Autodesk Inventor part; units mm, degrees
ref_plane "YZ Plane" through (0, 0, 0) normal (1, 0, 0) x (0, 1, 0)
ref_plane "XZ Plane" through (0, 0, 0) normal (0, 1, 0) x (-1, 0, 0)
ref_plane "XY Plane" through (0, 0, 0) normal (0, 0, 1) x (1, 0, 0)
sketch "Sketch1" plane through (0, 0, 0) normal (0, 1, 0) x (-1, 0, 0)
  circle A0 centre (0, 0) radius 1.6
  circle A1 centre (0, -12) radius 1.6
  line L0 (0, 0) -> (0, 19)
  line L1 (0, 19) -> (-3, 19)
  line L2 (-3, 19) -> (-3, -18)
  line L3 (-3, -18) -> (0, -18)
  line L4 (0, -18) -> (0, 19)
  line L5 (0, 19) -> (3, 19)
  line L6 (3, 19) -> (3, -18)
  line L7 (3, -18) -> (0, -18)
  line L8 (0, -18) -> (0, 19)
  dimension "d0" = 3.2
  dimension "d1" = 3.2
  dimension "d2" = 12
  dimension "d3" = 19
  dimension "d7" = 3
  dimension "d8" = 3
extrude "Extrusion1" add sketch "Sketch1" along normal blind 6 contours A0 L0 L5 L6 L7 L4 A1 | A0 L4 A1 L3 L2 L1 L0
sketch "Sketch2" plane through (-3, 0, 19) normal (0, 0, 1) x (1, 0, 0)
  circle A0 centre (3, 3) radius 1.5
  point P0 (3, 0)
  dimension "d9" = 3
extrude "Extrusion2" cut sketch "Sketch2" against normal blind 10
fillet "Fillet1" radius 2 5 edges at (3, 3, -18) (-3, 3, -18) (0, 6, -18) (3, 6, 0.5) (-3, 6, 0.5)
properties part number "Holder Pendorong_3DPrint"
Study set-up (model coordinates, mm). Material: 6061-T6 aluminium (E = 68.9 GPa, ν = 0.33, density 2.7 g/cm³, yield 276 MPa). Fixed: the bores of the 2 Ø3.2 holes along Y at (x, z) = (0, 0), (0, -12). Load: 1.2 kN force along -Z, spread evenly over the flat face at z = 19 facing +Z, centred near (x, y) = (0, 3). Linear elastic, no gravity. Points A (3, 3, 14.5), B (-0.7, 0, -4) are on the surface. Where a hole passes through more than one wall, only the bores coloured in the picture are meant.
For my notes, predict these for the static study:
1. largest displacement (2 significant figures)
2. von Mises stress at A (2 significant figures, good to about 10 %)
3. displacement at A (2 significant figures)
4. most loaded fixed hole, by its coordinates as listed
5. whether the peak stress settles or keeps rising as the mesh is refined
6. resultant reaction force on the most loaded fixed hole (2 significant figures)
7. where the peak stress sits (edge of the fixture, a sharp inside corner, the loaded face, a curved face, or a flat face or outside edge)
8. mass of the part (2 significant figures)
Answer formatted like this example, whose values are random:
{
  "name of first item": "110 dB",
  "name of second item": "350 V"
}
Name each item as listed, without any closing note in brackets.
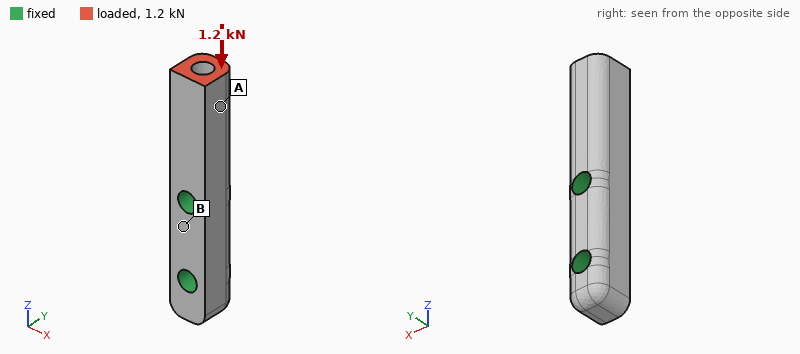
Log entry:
{
  "largest displacement": "11 µm",
  "von Mises stress at A": "44 MPa",
  "displacement at A": "7.9 µm",
  "most loaded fixed hole, by its coordinates as listed": "(0, 0)",
  "whether the peak stress settles or keeps rising as the mesh is refined": "keeps rising",
  "resultant reaction force on the most loaded fixed hole": "1.2 kN",
  "where the peak stress sits": "edge of the fixture",
  "mass of the part": "2.9 g"
}
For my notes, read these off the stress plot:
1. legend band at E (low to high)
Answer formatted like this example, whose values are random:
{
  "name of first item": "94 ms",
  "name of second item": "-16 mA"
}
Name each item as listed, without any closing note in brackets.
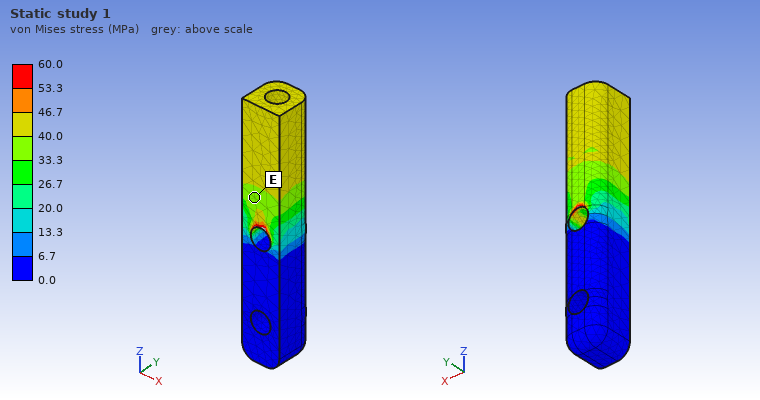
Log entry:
{
  "legend band at E": "33.3 to 40.0 MPa"
}
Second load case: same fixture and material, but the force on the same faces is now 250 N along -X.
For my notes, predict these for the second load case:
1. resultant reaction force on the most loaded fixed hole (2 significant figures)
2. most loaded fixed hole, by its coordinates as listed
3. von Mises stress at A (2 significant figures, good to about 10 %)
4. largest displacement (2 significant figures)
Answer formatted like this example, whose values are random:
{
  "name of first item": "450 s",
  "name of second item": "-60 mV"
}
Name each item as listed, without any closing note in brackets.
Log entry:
{
  "resultant reaction force on the most loaded fixed hole": "300 N",
  "most loaded fixed hole, by its coordinates as listed": "(0, 0)",
  "von Mises stress at A": "36 MPa",
  "largest displacement": "98 µm"
}
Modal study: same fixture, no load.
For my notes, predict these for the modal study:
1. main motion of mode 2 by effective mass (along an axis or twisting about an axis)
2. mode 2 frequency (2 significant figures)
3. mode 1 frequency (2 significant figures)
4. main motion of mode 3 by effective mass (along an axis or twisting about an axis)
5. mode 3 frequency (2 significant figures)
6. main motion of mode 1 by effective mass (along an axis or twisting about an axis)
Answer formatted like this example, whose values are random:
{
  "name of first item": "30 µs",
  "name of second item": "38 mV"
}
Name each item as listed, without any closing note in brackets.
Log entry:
{
  "main motion of mode 2 by effective mass": "along Y",
  "mode 2 frequency": "15 kHz",
  "mode 1 frequency": "14 kHz",
  "main motion of mode 3 by effective mass": "twisting about Z",
  "mode 3 frequency": "41 kHz",
  "main motion of mode 1 by effective mass": "along X"
}
